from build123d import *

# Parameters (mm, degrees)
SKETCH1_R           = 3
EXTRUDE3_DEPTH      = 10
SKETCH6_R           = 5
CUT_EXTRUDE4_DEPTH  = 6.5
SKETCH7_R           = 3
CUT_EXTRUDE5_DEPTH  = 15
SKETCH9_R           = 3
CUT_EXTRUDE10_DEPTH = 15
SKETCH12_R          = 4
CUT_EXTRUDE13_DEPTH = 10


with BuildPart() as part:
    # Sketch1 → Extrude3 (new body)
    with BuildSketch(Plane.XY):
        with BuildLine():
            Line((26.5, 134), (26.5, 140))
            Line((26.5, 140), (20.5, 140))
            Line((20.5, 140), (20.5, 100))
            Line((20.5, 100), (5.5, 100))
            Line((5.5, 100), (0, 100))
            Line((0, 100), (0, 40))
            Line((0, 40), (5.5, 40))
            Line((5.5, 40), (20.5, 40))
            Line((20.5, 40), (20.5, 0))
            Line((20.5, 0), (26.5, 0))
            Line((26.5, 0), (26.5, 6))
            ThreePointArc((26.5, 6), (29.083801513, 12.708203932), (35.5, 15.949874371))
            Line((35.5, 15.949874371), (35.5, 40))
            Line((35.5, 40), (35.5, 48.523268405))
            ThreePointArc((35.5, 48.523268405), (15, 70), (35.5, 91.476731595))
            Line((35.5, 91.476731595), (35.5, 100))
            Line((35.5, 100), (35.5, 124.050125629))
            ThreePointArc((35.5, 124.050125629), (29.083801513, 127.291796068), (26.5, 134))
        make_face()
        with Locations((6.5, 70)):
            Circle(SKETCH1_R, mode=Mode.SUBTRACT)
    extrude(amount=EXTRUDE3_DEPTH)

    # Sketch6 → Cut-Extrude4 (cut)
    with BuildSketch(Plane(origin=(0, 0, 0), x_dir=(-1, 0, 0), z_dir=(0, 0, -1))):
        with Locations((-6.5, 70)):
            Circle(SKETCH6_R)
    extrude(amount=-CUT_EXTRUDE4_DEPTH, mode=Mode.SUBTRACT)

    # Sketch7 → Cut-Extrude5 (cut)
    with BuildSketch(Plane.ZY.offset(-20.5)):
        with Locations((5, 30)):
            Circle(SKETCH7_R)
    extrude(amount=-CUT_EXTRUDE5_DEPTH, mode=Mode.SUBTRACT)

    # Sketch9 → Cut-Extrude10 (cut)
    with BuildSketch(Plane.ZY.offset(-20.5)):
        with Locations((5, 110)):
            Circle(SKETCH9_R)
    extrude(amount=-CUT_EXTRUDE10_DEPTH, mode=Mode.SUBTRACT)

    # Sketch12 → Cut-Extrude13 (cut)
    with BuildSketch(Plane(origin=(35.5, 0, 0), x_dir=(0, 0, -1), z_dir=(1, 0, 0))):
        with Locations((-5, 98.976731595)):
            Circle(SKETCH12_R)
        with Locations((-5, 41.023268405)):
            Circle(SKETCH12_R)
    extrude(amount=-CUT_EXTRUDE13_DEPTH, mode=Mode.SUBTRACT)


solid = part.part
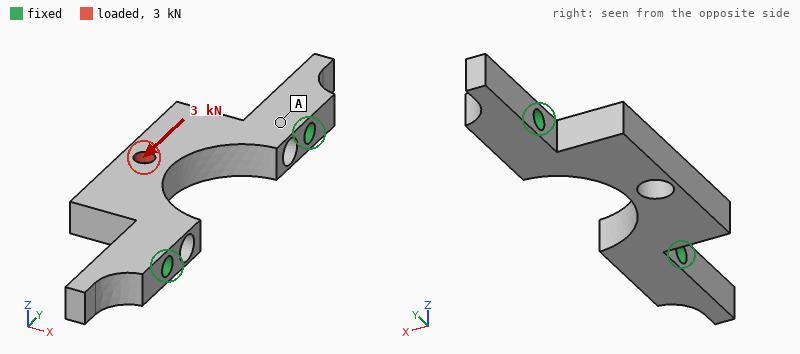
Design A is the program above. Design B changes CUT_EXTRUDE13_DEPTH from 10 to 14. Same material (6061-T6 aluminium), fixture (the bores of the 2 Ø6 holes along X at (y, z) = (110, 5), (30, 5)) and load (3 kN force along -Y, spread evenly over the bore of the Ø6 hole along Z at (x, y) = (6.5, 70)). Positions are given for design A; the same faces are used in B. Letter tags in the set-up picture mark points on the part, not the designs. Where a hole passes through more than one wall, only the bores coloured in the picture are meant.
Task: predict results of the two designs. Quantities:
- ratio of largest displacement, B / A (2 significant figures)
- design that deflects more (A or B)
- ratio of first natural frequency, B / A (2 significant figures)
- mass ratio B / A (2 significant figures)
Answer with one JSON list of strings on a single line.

["1.2", "B", "0.94", "0.98"]
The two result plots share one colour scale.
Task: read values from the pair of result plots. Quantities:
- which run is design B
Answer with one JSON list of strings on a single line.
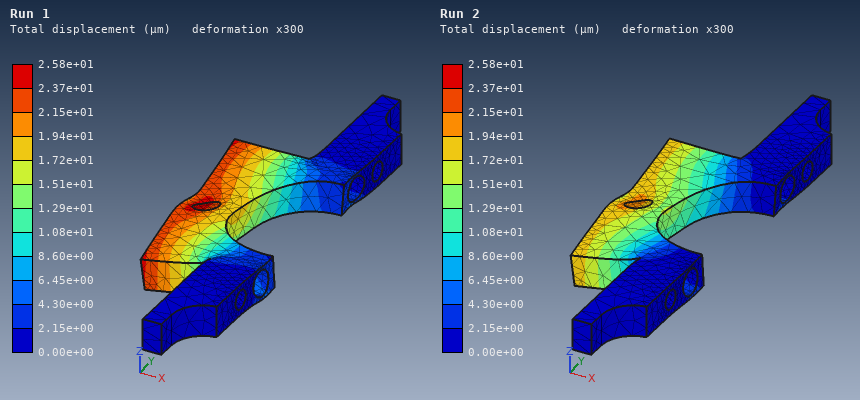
["Run 1"]
